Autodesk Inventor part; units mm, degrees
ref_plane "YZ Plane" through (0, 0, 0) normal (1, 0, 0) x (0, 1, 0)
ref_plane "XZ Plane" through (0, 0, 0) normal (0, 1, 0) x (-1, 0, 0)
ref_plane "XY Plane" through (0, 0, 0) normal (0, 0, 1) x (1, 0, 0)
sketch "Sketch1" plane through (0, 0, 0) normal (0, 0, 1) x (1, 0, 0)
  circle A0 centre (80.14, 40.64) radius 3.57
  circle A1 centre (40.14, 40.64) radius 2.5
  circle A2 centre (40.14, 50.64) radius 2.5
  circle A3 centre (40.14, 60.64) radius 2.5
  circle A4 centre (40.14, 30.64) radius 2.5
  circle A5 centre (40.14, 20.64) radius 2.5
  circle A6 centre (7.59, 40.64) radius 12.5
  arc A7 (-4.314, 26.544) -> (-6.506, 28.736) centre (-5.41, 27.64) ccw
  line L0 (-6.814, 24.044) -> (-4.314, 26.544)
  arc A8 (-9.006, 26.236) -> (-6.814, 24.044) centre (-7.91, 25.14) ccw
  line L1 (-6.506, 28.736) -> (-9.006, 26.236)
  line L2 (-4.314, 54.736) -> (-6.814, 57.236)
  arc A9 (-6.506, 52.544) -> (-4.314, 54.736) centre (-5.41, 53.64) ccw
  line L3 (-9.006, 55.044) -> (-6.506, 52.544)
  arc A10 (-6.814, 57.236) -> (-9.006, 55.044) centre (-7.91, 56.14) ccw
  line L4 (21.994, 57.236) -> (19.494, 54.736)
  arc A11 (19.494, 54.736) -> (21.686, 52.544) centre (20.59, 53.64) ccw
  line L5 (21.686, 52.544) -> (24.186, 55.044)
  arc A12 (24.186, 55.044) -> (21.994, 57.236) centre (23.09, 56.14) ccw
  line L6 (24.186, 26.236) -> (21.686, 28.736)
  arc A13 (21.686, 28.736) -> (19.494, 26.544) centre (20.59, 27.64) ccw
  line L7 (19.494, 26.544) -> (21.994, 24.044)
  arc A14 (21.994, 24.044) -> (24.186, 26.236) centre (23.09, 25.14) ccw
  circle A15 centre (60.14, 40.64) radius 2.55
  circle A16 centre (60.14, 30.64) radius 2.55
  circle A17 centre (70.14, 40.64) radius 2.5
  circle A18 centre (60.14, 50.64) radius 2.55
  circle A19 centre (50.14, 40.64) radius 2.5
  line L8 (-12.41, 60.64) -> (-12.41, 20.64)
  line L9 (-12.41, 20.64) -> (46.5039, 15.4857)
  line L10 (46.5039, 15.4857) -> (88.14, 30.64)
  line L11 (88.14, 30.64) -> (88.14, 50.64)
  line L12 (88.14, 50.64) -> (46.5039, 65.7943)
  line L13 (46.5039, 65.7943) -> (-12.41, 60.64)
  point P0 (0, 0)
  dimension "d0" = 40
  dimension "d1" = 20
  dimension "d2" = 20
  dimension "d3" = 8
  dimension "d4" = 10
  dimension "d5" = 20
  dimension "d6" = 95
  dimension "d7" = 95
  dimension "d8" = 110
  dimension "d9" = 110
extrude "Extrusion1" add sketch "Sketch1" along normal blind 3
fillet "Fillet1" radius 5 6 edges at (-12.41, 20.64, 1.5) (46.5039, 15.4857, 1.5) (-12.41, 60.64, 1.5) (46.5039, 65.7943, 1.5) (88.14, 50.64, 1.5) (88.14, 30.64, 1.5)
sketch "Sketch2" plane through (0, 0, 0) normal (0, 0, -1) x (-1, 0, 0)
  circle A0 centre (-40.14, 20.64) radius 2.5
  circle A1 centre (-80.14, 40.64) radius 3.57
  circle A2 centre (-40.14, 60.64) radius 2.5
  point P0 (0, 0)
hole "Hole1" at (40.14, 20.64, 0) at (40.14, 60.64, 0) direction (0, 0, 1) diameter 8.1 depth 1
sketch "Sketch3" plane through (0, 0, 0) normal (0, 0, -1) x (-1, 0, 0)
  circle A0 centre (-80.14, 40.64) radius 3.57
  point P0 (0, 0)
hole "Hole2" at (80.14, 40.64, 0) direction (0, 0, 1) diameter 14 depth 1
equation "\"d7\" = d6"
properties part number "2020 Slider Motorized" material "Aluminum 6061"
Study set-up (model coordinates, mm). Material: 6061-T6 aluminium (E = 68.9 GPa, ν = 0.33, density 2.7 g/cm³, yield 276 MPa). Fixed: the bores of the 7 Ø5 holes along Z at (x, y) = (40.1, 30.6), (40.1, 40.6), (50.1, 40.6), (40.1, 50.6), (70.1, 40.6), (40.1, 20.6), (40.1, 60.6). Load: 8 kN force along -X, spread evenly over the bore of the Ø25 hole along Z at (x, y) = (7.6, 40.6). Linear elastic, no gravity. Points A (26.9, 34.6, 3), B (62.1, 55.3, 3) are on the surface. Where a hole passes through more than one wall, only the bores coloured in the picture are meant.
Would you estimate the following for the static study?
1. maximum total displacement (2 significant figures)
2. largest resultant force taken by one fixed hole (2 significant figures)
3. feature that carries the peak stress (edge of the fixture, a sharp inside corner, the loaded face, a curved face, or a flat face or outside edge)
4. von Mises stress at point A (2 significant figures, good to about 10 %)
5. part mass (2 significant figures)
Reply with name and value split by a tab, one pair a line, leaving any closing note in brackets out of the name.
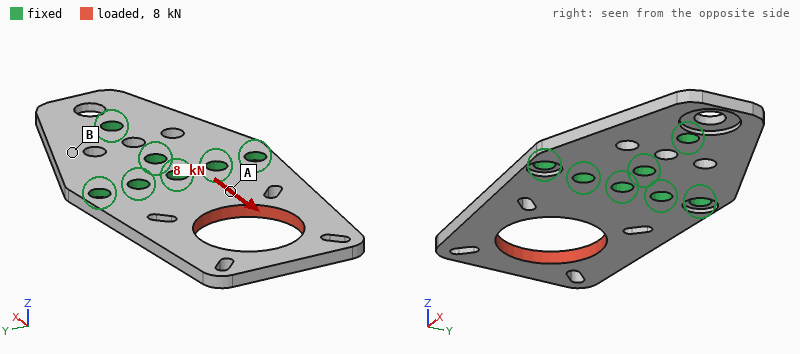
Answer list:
maximum total displacement	0.11 mm
largest resultant force taken by one fixed hole	2.1 kN
feature that carries the peak stress	a curved face
von Mises stress at point A	53 MPa
part mass	26 g
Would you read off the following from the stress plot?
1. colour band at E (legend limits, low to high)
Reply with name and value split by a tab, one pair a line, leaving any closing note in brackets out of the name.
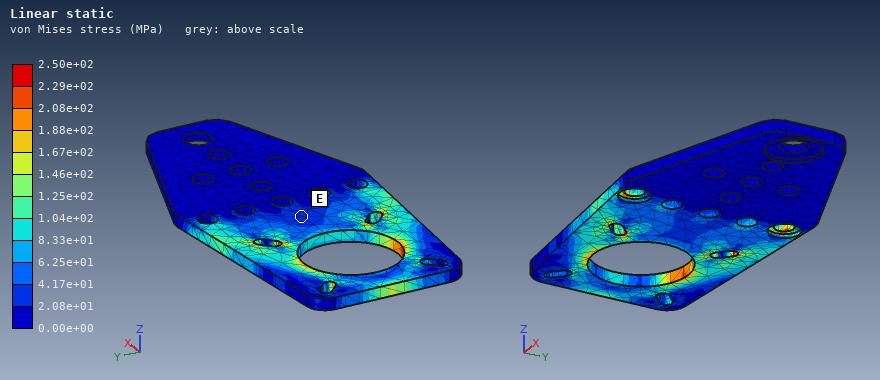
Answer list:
colour band at E	2.08e+01 to 4.17e+01 MPa
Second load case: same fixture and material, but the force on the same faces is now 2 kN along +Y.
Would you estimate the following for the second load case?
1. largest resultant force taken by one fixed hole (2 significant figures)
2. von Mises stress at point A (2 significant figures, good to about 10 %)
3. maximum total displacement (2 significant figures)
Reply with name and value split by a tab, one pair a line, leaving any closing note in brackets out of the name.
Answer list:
largest resultant force taken by one fixed hole	1.3 kN
von Mises stress at point A	46 MPa
maximum total displacement	0.10 mm
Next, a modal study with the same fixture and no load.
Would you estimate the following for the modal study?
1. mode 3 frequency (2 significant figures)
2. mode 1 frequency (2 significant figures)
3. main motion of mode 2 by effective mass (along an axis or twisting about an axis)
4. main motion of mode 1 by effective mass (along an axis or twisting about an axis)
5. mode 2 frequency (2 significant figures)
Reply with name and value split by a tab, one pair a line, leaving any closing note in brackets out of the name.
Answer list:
mode 3 frequency	5300 Hz
mode 1 frequency	1000 Hz
main motion of mode 2 by effective mass	twisting about X
main motion of mode 1 by effective mass	along Z
mode 2 frequency	2400 Hz
